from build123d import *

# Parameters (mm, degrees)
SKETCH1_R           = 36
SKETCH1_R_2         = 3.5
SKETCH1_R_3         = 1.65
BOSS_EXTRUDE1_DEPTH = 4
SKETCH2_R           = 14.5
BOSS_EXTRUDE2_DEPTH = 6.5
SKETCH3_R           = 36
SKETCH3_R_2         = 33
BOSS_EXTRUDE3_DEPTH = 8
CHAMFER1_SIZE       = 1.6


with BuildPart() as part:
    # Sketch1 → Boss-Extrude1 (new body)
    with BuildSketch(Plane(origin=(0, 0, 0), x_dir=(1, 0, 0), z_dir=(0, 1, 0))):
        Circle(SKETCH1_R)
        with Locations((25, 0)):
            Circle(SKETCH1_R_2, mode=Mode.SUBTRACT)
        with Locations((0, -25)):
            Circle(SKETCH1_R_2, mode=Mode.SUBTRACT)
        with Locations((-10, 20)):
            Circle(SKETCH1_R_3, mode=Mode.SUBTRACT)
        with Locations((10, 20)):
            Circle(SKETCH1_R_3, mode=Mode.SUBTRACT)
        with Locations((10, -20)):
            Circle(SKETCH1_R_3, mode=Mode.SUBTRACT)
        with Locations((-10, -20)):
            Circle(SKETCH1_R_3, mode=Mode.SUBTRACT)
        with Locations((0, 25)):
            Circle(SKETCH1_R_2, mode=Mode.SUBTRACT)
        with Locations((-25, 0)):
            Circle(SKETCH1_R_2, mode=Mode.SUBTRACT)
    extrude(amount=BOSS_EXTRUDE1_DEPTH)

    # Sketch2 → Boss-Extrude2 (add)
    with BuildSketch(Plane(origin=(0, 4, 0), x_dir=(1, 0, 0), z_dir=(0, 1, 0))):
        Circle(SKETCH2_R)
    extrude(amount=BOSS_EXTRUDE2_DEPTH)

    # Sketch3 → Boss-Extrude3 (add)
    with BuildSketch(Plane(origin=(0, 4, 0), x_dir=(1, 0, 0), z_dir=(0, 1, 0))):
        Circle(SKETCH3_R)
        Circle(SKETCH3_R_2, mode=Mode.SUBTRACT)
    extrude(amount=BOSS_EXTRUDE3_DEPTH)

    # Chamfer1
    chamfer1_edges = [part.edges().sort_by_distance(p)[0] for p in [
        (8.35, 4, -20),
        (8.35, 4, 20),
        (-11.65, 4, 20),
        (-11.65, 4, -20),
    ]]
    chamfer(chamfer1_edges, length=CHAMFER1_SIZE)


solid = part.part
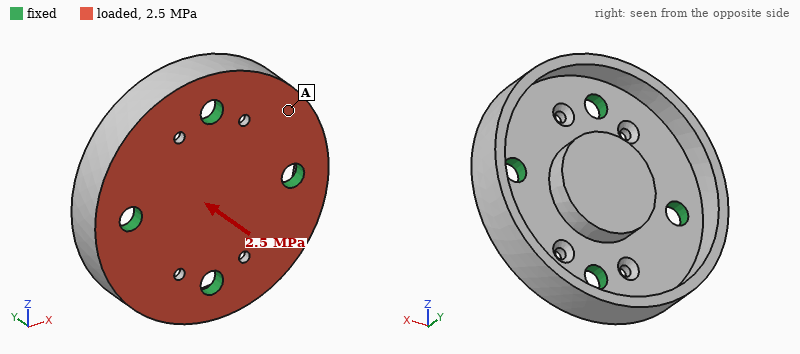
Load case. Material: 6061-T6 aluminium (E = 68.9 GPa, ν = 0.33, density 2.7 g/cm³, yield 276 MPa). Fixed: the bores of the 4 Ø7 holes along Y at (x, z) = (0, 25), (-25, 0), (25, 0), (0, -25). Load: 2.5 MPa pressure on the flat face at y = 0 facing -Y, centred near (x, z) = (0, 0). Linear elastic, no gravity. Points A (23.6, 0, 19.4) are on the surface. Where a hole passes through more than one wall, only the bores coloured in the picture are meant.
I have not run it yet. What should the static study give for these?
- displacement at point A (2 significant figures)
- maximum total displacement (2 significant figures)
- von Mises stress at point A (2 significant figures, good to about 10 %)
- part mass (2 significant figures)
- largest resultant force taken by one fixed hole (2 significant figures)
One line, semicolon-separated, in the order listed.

20 µm; 24 µm; 17 MPa; 67 g; 2.4 kN
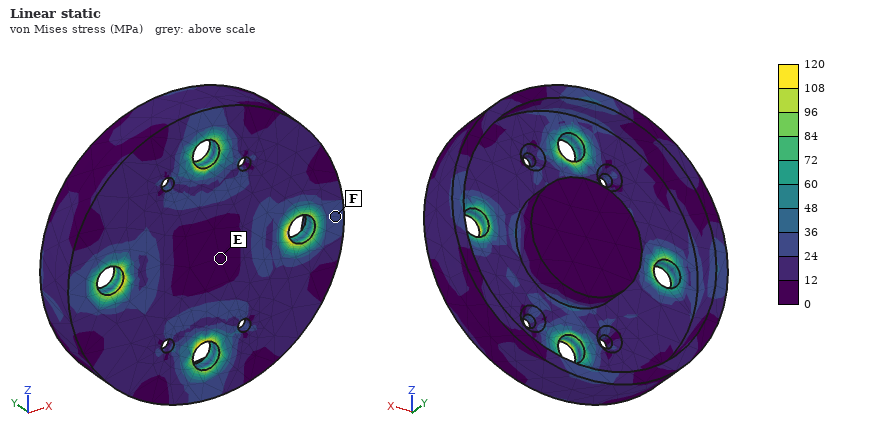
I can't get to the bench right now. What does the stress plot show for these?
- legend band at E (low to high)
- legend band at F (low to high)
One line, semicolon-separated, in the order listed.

0 to 12 MPa; 24 to 36 MPa
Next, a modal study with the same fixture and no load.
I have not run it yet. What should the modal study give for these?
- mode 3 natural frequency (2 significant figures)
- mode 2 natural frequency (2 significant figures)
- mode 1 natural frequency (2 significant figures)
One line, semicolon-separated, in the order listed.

11 kHz; 11 kHz; 8100 Hz
